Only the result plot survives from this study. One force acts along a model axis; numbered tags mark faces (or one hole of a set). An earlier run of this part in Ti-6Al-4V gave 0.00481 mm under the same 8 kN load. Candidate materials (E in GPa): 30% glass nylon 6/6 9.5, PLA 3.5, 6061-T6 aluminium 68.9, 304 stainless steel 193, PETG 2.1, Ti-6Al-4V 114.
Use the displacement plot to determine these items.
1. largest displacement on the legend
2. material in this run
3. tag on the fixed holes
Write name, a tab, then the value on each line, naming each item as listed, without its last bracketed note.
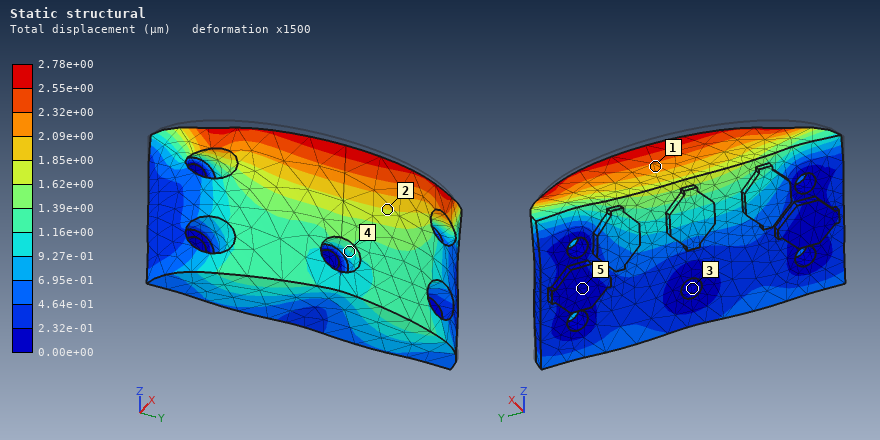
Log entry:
largest displacement on the legend	2.78e+00 µm
material in this run	304 stainless steel
tag on the fixed holes	3
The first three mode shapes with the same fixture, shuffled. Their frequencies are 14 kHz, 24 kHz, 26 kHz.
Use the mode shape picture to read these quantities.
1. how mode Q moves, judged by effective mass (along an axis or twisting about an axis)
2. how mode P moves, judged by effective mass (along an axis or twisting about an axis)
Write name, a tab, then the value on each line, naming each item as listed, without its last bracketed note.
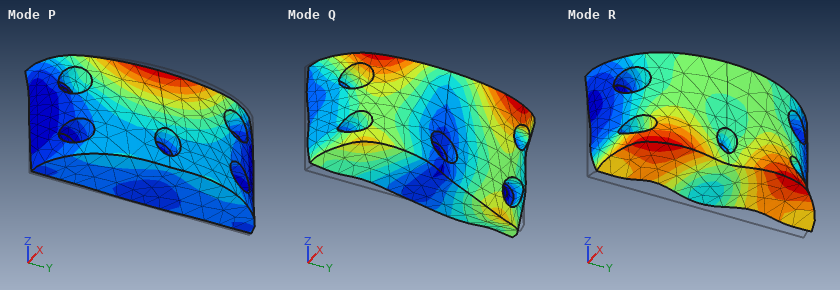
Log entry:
how mode Q moves, judged by effective mass	along Y
how mode P moves, judged by effective mass	along X
